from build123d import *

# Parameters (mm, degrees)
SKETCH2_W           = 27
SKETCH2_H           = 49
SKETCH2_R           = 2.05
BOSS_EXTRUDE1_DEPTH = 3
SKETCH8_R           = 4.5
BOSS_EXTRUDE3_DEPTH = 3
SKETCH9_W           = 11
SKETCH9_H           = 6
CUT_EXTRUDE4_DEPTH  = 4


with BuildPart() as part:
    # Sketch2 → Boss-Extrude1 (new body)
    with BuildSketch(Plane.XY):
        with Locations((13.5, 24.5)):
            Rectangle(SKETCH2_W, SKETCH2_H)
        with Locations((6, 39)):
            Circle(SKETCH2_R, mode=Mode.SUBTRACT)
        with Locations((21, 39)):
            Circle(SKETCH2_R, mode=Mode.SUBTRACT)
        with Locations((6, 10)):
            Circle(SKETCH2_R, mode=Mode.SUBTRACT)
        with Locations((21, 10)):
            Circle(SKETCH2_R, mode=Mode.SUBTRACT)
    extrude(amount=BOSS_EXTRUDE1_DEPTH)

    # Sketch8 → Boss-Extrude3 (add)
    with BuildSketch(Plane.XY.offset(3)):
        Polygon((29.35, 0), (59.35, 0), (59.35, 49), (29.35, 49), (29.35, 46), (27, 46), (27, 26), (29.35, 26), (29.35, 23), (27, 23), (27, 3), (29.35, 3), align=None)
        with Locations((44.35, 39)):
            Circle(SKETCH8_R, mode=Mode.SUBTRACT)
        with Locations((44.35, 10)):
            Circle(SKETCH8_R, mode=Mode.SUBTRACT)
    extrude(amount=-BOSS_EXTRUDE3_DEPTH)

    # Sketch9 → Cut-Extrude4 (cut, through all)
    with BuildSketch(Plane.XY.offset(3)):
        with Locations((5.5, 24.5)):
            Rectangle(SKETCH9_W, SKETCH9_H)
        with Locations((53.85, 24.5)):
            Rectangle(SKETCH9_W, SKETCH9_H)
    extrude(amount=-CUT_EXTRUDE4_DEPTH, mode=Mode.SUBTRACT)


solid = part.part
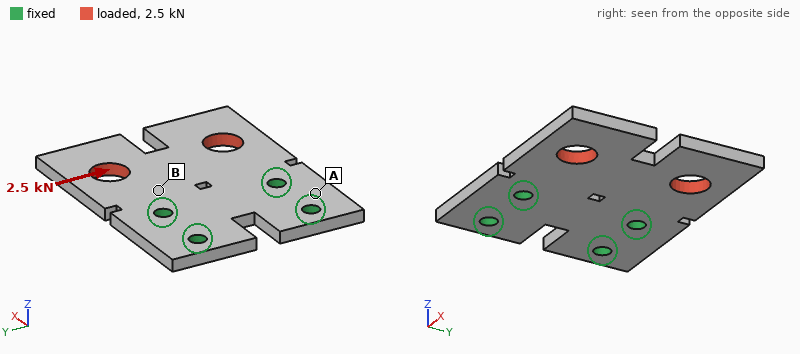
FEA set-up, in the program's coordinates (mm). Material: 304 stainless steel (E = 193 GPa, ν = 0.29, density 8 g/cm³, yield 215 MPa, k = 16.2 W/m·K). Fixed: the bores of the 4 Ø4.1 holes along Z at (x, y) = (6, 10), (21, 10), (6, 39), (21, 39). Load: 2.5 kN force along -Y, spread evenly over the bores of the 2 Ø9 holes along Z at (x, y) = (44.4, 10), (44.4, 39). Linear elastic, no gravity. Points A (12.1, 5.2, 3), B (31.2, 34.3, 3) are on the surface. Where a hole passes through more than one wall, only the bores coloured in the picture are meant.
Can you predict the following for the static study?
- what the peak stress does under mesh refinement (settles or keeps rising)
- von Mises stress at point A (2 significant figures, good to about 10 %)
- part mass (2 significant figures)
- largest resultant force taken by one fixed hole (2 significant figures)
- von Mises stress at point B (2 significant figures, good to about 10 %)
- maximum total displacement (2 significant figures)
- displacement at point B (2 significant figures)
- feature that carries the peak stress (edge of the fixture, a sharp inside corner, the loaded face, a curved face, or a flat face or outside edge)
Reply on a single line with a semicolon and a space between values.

keeps rising; 15 MPa; 62 g; 1.9 kN; 50 MPa; 16 µm; 4.1 µm; edge of the fixture
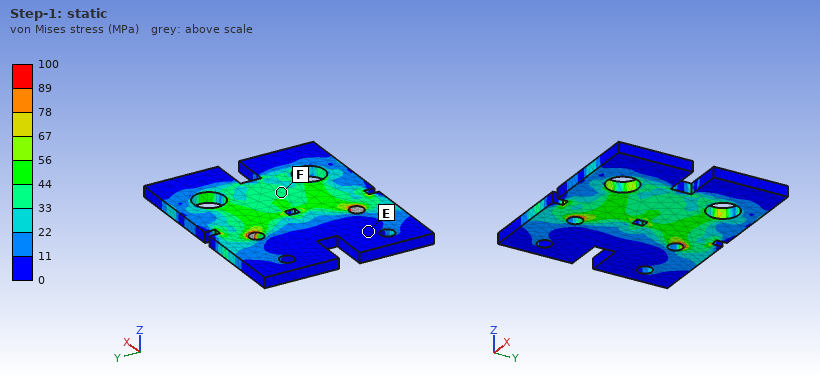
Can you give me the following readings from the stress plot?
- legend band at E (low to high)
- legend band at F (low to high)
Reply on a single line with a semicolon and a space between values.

0 to 11 MPa; 33 to 44 MPa
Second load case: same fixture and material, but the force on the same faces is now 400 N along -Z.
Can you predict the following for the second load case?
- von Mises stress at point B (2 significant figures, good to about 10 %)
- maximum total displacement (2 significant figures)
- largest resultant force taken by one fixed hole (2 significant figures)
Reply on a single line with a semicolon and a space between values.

71 MPa; 0.17 mm; 290 N
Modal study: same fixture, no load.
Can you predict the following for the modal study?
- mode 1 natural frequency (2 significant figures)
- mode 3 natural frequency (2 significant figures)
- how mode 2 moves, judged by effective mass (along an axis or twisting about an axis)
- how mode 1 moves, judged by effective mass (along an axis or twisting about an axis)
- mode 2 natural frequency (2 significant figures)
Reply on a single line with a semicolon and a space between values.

1700 Hz; 6700 Hz; twisting about X; along Z; 2800 Hz
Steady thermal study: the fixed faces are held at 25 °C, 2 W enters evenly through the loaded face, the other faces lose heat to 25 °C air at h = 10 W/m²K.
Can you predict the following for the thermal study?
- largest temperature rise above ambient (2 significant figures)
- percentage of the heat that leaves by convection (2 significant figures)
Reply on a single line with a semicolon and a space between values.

21 K; 25 %
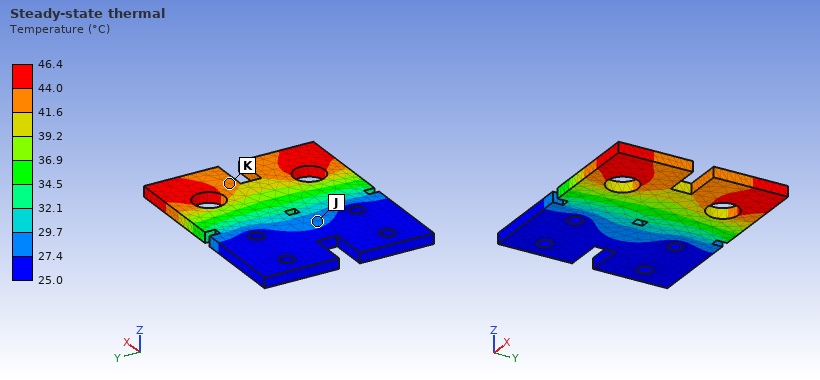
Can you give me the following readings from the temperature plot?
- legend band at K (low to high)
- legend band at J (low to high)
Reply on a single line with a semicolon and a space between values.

41.6 to 44.0 °C; 27.4 to 29.7 °C
